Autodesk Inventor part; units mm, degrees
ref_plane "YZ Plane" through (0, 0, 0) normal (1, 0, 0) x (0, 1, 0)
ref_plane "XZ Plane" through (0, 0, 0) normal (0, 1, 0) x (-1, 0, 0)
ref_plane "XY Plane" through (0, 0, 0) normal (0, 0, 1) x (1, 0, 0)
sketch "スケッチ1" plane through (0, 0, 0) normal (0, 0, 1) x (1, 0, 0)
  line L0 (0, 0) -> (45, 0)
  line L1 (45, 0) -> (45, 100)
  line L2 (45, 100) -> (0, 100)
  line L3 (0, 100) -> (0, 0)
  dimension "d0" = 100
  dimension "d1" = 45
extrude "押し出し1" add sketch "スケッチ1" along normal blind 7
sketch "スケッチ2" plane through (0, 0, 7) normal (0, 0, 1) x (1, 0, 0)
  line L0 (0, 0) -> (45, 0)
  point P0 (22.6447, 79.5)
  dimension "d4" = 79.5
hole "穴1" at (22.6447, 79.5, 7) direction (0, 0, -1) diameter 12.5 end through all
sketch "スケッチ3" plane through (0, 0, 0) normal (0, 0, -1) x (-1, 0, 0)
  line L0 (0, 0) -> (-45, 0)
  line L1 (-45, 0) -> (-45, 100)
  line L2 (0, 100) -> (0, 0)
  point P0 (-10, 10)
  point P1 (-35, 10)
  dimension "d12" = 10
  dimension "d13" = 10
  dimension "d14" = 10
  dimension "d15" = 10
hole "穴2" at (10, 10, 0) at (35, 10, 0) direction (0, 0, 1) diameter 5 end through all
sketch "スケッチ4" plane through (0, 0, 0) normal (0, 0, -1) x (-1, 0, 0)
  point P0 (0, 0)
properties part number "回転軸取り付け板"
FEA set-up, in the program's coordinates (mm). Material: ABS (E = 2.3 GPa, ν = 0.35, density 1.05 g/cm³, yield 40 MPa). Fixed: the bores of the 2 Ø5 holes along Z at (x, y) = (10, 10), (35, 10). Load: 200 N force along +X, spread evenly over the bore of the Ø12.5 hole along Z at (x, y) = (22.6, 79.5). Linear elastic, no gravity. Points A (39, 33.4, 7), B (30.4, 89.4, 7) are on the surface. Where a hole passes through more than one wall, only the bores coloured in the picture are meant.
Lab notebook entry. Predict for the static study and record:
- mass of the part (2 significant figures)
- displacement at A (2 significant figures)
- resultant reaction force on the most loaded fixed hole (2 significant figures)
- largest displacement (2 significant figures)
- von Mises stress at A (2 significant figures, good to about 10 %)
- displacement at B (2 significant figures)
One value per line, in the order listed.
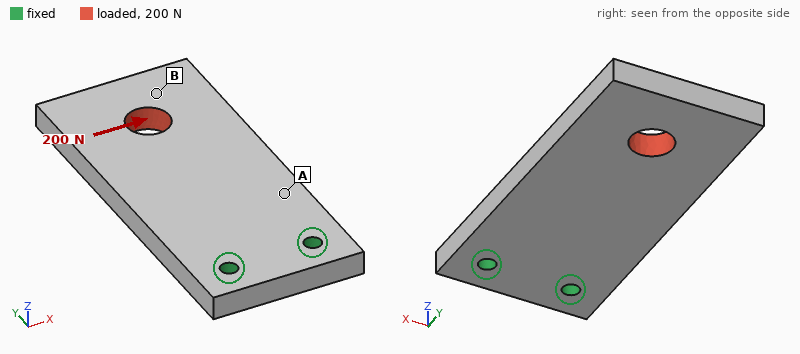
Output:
32 g
0.080 mm
510 N
0.40 mm
2.9 MPa
0.34 mm
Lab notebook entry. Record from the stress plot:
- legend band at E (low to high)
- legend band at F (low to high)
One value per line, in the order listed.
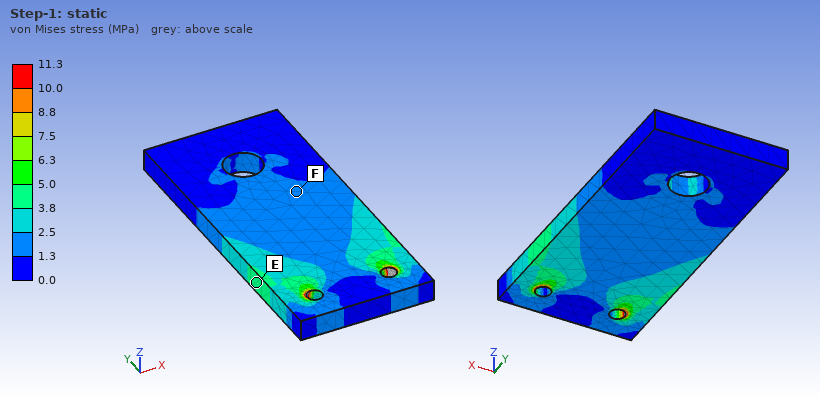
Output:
3.8 to 5.0 MPa
1.3 to 2.5 MPa
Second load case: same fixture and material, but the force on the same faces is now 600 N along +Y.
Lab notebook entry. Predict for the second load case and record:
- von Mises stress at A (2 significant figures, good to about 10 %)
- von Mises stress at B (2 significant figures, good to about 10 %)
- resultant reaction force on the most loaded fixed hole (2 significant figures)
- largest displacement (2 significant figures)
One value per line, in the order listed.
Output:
1.9 MPa
1.7 MPa
310 N
82 µm
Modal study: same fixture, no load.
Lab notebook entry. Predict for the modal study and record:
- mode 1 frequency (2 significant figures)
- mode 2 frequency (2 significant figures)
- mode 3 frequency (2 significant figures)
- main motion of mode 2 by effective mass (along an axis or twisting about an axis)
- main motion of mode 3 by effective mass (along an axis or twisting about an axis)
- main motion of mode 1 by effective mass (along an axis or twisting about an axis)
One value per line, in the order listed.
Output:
210 Hz
820 Hz
1100 Hz
twisting about Y
along X
along Z
